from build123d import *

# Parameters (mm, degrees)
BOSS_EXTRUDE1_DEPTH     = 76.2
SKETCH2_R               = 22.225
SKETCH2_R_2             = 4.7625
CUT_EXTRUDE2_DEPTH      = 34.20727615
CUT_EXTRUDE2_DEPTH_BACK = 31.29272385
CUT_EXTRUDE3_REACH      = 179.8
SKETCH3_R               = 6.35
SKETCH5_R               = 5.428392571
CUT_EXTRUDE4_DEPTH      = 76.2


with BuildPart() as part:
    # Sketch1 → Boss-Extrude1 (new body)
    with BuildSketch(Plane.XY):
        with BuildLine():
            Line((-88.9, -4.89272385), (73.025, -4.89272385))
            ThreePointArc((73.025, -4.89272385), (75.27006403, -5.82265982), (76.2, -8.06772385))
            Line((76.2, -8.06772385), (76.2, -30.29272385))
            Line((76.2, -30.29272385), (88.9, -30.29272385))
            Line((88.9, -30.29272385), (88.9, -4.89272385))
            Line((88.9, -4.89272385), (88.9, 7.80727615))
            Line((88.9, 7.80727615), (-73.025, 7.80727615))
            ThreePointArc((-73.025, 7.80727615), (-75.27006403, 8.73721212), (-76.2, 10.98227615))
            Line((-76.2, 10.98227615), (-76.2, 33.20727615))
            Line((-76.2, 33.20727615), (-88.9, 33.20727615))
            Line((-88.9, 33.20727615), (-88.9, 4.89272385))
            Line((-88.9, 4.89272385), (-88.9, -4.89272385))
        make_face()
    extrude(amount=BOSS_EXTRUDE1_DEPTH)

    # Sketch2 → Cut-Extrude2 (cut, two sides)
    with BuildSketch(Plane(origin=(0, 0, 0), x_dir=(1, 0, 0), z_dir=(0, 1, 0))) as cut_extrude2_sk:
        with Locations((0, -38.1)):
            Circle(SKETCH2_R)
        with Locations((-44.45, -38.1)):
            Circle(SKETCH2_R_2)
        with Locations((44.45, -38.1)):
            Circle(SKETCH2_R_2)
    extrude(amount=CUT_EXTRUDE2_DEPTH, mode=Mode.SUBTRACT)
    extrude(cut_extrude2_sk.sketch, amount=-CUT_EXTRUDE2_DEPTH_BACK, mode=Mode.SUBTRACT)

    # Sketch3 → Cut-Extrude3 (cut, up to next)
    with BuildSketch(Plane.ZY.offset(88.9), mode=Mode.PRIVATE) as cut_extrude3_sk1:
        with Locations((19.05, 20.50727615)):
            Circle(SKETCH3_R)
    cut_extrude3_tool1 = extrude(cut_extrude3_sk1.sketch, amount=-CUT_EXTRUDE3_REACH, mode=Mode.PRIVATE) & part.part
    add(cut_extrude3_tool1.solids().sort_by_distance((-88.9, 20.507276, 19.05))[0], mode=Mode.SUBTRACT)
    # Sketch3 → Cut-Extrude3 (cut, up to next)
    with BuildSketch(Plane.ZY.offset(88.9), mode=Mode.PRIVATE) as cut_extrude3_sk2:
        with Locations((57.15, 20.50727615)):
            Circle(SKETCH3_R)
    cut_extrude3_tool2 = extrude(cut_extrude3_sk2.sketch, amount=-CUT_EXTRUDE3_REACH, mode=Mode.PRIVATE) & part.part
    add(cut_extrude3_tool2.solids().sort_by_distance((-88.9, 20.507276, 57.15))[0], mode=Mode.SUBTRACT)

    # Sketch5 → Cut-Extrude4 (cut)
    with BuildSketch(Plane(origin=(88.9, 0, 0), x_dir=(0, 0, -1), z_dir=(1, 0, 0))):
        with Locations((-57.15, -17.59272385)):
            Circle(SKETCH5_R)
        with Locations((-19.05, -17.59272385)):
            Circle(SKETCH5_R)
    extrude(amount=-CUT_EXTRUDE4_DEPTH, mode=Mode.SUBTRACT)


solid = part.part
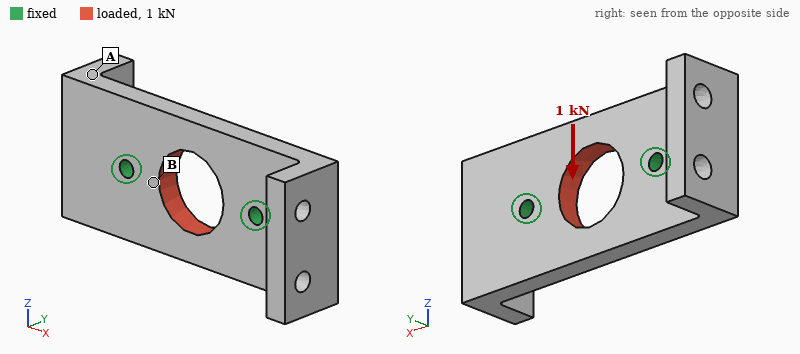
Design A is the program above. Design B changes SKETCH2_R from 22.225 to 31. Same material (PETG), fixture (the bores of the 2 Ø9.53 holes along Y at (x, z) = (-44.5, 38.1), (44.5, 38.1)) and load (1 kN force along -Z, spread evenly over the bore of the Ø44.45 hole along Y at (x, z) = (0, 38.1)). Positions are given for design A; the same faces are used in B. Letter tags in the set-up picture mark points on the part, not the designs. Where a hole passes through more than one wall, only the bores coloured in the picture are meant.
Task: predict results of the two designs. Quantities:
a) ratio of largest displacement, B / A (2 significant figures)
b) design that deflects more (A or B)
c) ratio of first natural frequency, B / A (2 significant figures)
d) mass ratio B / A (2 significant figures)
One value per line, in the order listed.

1.6
B
0.98
0.90
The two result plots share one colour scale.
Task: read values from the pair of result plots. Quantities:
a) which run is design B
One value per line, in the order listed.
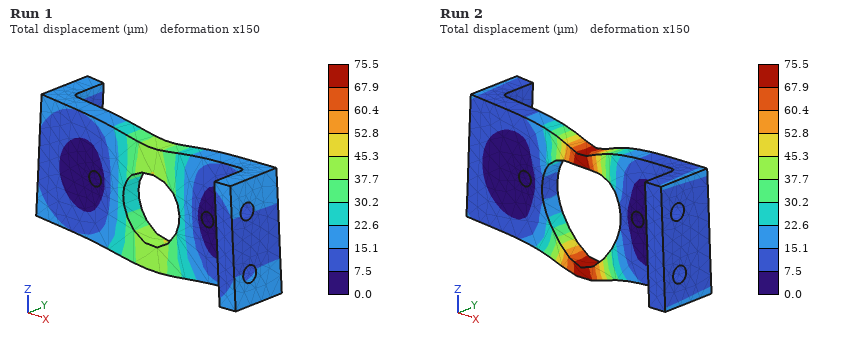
Run 2
